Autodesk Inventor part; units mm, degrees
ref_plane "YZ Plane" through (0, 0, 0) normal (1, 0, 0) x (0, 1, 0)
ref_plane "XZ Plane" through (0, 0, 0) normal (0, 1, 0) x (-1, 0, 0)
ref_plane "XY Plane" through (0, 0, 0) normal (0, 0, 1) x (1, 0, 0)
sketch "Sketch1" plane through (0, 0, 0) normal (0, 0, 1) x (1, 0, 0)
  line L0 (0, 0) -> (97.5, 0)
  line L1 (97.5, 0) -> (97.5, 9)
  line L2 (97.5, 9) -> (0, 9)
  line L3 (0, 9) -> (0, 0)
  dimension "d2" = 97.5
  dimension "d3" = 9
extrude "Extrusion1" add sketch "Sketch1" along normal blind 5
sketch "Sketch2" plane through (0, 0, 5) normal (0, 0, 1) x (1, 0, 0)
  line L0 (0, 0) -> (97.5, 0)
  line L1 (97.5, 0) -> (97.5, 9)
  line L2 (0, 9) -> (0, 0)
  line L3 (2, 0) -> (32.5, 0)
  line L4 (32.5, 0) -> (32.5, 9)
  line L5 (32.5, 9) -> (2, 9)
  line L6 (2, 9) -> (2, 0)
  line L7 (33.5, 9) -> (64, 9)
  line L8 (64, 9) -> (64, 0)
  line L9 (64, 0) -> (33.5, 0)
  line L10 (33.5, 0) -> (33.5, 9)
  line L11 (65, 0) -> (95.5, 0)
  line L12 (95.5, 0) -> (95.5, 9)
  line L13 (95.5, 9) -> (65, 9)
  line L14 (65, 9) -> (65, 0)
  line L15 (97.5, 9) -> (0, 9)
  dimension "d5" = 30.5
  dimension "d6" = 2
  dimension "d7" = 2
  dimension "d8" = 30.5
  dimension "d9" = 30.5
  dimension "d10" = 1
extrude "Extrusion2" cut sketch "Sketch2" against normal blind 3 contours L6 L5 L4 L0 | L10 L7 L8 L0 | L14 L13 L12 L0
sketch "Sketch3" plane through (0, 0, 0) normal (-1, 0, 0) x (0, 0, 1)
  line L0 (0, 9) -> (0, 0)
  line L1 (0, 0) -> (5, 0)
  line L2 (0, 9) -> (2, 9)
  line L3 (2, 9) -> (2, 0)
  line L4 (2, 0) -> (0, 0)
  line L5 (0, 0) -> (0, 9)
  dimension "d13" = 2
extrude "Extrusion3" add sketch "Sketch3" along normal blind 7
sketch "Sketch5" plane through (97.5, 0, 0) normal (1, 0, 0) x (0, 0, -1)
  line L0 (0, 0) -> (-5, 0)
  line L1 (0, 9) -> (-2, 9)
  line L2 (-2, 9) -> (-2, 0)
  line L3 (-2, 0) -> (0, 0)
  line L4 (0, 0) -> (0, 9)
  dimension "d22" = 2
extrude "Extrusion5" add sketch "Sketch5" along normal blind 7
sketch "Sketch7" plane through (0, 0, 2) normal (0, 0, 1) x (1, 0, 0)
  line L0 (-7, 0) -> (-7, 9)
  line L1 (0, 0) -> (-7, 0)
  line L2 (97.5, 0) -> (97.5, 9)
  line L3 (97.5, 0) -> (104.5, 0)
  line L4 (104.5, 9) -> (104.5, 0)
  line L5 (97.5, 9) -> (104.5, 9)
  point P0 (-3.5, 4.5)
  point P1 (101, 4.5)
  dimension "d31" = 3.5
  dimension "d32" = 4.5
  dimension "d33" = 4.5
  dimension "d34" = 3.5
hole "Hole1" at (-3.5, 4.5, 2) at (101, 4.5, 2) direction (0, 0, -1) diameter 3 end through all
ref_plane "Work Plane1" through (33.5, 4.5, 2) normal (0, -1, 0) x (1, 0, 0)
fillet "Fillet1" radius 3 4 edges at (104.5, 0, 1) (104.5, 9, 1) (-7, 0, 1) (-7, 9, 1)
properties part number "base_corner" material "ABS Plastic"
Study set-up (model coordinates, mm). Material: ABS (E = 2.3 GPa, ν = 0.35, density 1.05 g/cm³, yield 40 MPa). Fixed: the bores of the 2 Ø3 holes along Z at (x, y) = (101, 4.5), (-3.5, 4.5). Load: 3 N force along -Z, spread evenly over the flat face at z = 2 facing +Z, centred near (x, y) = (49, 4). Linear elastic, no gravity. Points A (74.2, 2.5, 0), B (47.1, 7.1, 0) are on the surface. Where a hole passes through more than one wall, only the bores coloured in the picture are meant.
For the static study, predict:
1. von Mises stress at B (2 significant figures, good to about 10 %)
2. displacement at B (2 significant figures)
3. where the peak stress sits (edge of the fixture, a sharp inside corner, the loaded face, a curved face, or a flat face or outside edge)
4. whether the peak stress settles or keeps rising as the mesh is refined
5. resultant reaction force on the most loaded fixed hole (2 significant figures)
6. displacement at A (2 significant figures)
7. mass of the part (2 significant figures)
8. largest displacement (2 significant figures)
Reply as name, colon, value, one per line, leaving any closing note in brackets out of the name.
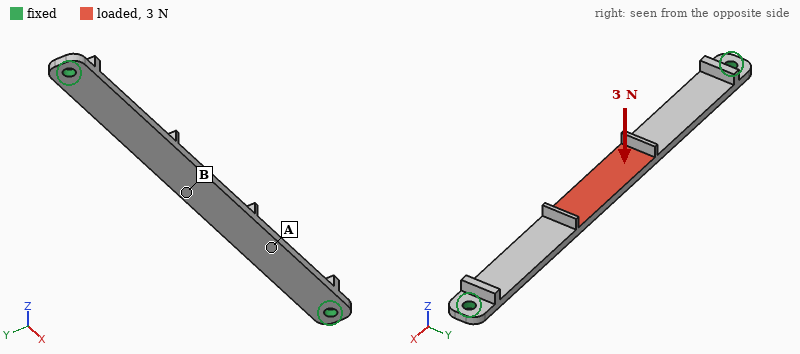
von Mises stress at B: 4.6 MPa
displacement at B: 1.1 mm
where the peak stress sits: edge of the fixture
whether the peak stress settles or keeps rising as the mesh is refined: keeps rising
resultant reaction force on the most loaded fixed hole: 1.5 N
displacement at A: 0.57 mm
mass of the part: 2.2 g
largest displacement: 1.1 mm
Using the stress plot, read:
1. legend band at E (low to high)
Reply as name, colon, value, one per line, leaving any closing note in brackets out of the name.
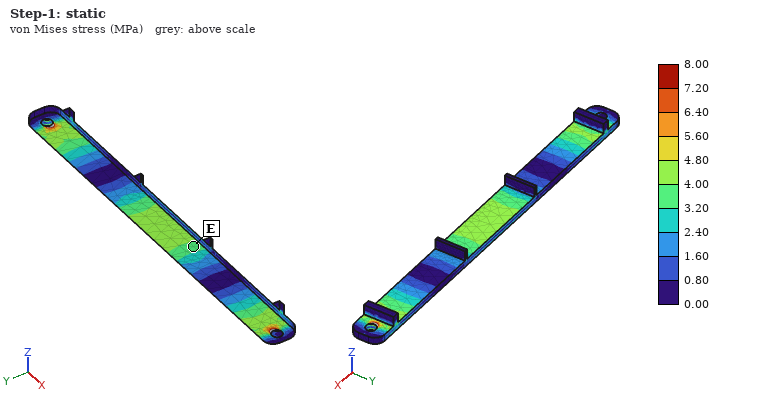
legend band at E: 3.20 to 4.00 MPa
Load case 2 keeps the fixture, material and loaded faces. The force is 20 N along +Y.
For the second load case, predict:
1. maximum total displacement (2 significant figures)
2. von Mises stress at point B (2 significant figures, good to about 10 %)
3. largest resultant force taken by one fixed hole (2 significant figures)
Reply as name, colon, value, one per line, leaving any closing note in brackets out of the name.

maximum total displacement: 0.55 mm
von Mises stress at point B: 4.6 MPa
largest resultant force taken by one fixed hole: 10 N
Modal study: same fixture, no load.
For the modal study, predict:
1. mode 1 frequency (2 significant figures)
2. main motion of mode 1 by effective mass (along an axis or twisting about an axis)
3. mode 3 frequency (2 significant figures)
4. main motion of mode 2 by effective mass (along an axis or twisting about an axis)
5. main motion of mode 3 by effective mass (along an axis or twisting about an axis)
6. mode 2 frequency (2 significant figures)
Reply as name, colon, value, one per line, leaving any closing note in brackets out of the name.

mode 1 frequency: 290 Hz
main motion of mode 1 by effective mass: along Z
mode 3 frequency: 1000 Hz
main motion of mode 2 by effective mass: twisting about Y
main motion of mode 3 by effective mass: along Y
mode 2 frequency: 790 Hz
